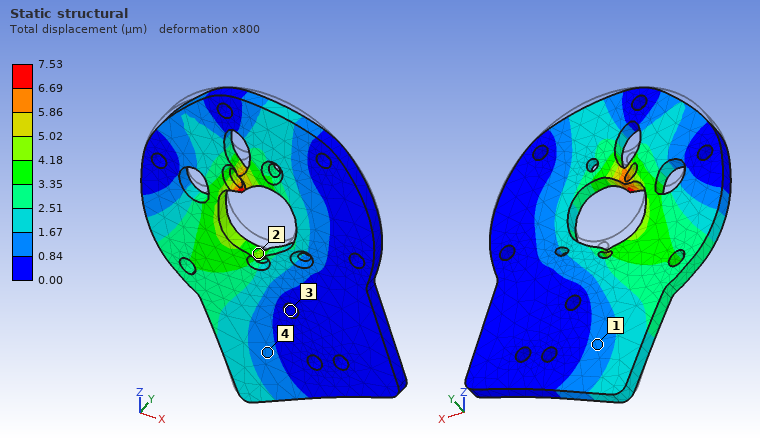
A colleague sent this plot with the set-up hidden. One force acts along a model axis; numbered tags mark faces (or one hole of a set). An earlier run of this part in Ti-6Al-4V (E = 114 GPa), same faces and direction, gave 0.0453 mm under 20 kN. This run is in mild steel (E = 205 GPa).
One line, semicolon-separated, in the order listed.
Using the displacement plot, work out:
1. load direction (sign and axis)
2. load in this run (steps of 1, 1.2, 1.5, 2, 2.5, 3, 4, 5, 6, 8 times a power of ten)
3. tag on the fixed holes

-Z; 6 kN; 3
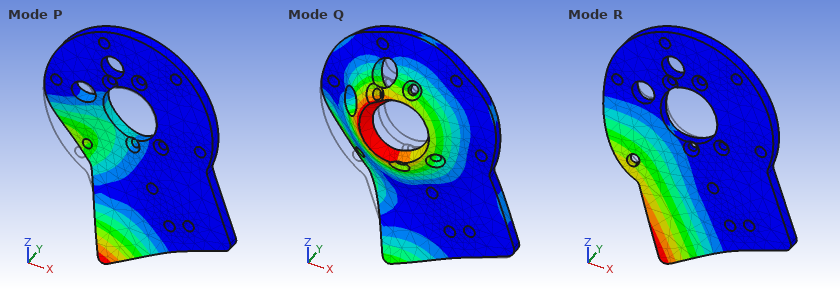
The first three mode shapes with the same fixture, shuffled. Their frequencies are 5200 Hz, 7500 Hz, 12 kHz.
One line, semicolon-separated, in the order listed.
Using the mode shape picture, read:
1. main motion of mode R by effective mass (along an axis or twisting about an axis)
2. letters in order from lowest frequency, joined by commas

along Y; R, P, Q
